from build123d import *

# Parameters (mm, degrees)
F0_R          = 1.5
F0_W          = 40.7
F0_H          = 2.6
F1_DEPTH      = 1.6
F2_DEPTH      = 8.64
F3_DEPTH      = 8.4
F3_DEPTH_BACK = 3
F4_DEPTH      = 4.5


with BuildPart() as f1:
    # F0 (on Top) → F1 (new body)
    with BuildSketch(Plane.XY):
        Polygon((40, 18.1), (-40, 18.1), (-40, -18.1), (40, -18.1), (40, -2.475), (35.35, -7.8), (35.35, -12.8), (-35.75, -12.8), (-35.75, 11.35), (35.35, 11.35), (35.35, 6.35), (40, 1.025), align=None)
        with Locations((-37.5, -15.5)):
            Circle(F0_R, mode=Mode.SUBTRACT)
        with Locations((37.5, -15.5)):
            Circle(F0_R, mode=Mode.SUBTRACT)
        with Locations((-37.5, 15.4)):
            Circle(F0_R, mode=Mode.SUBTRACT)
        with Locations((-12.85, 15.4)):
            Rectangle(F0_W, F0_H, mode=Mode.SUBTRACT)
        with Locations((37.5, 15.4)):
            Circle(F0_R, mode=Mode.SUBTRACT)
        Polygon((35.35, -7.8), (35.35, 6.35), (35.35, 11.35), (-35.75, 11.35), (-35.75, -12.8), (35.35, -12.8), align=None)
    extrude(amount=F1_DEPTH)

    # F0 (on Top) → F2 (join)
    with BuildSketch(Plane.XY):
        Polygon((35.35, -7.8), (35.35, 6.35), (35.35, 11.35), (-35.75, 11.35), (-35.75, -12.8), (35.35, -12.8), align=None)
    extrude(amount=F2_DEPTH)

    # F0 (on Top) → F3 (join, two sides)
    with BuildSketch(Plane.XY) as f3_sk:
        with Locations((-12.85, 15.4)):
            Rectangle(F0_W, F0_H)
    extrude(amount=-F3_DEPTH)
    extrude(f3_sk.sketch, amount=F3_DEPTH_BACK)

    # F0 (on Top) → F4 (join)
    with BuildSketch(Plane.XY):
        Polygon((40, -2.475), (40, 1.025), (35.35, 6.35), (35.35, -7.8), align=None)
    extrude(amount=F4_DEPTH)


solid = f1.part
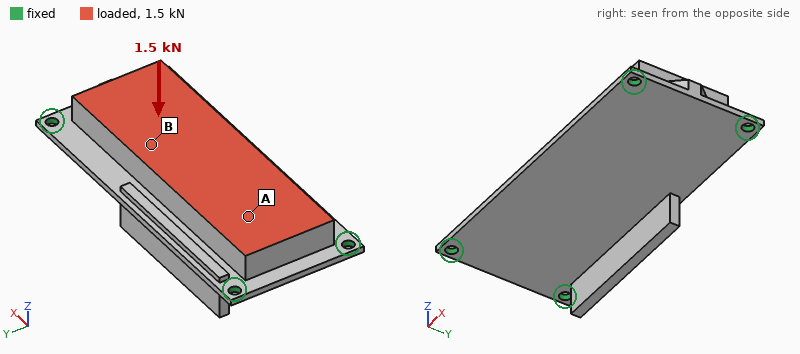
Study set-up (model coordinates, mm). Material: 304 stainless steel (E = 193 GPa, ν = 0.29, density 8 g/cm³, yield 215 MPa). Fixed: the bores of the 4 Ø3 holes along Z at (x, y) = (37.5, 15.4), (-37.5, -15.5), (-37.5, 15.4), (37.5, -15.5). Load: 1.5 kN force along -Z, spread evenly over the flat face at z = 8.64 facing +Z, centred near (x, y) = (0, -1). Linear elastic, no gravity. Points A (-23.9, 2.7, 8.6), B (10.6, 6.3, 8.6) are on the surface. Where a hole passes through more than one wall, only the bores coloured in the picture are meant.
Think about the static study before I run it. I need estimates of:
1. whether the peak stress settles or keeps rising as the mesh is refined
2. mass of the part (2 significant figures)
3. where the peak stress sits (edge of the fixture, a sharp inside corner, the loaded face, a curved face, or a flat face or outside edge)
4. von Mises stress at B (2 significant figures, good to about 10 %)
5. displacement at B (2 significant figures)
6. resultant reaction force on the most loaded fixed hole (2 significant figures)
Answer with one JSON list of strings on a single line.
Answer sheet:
["keeps rising", "140 g", "edge of the fixture", "32 MPa", "24 µm", "700 N"]
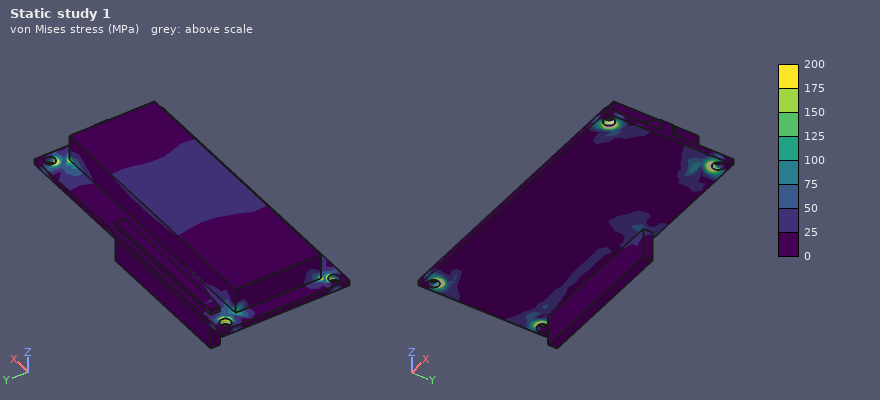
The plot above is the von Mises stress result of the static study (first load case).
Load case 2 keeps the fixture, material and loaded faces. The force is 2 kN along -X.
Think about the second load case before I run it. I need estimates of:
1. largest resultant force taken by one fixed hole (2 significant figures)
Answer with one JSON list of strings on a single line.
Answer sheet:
["570 N"]
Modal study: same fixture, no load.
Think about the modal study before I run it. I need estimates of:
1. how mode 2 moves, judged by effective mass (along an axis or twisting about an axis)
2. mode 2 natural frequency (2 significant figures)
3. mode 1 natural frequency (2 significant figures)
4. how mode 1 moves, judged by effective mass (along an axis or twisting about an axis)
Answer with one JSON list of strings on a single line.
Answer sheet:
["twisting about X", "6500 Hz", "3700 Hz", "along Z"]
